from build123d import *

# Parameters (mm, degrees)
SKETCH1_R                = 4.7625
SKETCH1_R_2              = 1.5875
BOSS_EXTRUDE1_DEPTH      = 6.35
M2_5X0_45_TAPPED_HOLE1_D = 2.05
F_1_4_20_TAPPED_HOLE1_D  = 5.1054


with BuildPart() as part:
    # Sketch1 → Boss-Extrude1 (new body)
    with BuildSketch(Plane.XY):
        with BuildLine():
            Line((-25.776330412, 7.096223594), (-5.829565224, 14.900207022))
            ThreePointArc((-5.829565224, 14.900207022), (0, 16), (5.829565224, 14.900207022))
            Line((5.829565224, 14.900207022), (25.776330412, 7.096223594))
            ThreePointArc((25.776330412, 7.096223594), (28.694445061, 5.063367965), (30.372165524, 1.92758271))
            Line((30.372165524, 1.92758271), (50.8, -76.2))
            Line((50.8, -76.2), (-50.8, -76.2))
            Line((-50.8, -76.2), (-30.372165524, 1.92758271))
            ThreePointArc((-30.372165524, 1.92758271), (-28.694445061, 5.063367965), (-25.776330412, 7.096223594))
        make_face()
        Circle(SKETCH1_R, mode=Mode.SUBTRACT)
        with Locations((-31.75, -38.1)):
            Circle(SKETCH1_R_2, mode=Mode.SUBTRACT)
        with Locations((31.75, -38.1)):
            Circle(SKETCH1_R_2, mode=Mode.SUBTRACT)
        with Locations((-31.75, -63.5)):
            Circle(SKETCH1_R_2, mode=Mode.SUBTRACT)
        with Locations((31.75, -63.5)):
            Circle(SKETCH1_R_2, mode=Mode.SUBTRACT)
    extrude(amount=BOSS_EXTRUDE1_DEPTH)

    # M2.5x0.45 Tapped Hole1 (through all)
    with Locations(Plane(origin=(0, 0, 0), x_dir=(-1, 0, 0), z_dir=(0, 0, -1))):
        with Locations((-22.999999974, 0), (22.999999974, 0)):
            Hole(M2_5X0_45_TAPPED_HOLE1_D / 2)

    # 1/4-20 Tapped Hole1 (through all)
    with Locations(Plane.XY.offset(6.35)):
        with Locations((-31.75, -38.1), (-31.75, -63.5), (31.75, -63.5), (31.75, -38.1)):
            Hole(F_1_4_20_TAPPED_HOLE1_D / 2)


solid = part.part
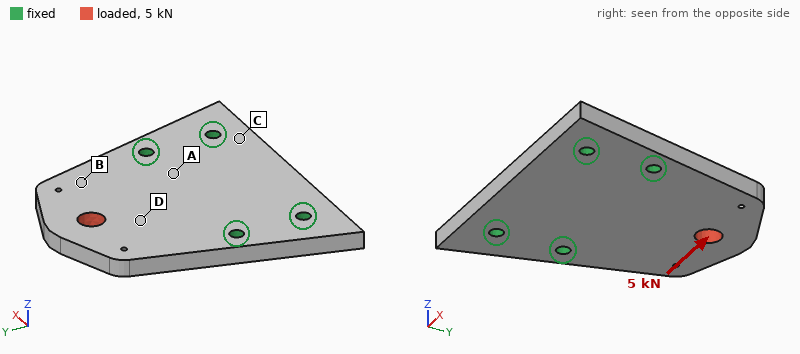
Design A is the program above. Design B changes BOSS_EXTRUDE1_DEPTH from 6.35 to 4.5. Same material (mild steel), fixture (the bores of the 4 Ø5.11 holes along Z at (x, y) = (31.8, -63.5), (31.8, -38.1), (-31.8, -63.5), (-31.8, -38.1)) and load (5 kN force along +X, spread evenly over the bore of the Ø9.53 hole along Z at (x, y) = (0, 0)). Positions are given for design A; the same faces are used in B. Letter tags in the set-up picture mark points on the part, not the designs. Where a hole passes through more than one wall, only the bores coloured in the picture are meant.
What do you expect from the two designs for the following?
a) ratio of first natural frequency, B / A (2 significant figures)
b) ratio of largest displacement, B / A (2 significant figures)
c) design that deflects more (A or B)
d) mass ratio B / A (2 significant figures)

0.73
1.4
B
0.71
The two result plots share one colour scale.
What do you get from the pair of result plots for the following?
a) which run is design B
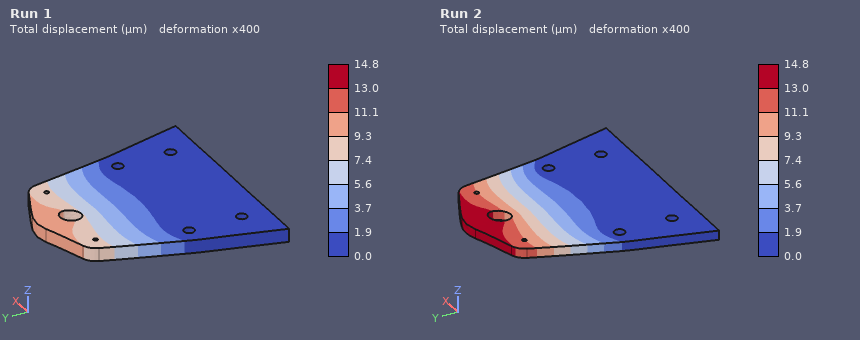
Run 2
